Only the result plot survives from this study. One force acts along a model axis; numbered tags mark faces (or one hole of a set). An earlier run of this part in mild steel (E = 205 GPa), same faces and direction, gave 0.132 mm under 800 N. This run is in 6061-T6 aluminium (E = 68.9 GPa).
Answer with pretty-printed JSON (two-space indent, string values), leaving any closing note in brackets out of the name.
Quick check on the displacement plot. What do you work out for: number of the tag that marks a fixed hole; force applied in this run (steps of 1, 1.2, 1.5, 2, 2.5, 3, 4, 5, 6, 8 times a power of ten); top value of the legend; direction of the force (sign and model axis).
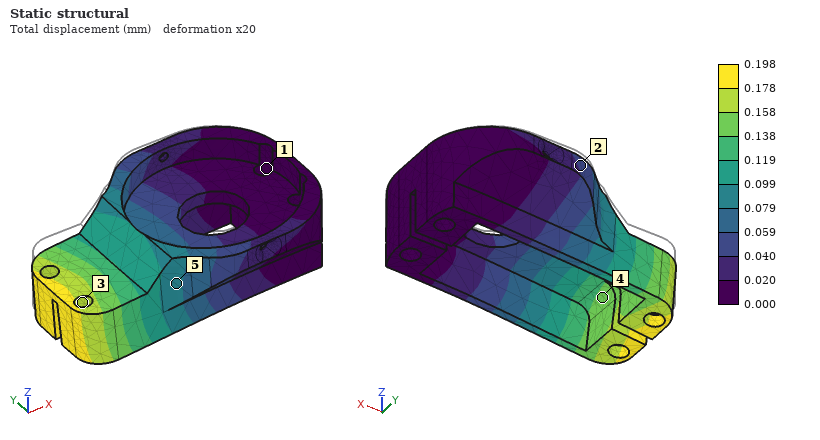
{
  "number of the tag that marks a fixed hole": "1",
  "force applied in this run": "400 N",
  "top value of the legend": "0.198 mm",
  "direction of the force": "-Z"
}
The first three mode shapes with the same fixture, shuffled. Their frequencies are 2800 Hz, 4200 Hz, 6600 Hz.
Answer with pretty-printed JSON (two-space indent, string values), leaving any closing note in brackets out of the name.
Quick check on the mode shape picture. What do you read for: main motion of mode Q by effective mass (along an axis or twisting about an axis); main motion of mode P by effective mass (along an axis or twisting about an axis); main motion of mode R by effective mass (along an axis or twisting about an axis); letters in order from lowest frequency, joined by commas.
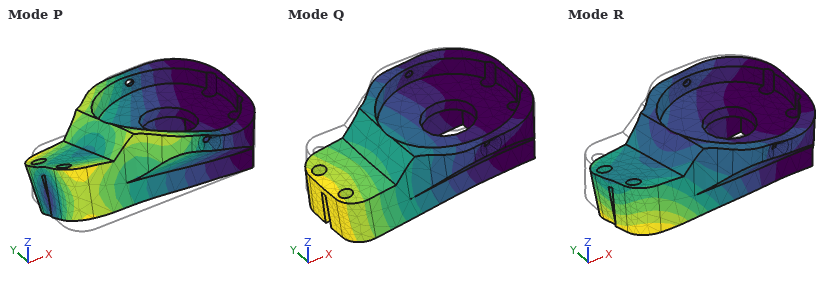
{
  "main motion of mode Q by effective mass": "along Z",
  "main motion of mode P by effective mass": "along Y",
  "main motion of mode R by effective mass": "along Y",
  "letters in order from lowest frequency, joined by commas": "Q, R, P"
}
